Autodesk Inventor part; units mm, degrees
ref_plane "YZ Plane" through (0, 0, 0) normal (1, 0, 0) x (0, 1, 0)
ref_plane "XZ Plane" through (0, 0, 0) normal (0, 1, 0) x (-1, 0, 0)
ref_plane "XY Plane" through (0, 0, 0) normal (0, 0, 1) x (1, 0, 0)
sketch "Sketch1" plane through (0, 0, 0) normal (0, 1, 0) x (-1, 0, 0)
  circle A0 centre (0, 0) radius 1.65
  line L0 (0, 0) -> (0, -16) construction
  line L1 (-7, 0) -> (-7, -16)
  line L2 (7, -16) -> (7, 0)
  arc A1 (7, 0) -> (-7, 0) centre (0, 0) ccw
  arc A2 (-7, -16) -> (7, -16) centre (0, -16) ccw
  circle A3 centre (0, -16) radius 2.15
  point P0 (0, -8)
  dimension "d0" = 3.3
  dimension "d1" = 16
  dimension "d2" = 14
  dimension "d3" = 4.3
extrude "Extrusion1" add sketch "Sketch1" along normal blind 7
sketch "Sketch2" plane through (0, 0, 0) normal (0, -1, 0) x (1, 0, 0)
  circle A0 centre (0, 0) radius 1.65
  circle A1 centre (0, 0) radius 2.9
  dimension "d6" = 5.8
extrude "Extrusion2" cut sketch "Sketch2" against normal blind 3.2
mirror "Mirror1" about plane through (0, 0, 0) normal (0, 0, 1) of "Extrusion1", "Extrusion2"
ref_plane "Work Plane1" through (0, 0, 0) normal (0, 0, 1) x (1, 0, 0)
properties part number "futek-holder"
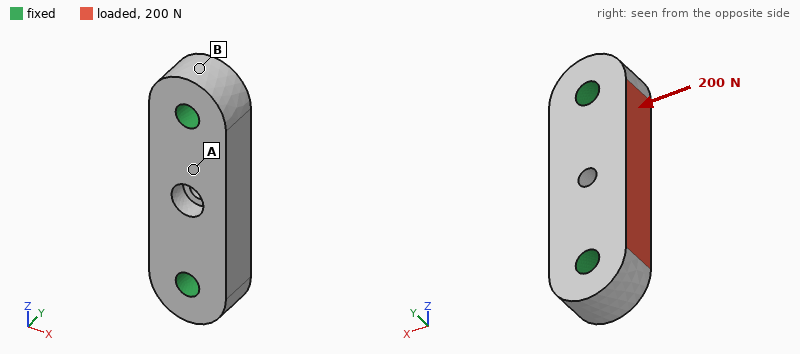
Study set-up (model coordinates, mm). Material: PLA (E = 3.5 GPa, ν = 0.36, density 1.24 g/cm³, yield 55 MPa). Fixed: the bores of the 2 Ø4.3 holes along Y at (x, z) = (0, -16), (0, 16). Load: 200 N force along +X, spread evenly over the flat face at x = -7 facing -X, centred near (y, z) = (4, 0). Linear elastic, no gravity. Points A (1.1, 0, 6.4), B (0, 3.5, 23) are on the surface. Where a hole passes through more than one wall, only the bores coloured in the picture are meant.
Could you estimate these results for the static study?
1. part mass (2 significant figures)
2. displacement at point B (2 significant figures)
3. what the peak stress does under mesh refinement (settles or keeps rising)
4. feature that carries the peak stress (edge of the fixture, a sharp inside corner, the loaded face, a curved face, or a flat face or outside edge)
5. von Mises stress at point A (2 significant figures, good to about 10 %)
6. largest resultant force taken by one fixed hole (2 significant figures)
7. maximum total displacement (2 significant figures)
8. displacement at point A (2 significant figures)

4.8 g
2.3 µm
keeps rising
edge of the fixture
1.1 MPa
100 N
14 µm
9.7 µm
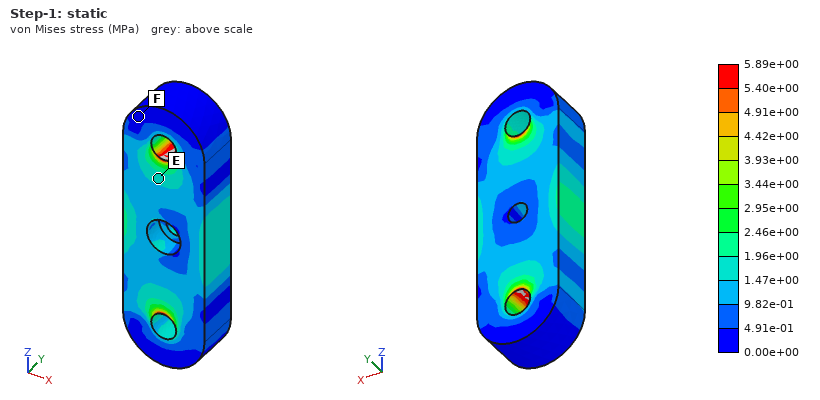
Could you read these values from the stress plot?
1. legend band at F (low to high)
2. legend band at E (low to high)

0.00e+00 to 4.91e-01 MPa
1.47e+00 to 1.96e+00 MPa
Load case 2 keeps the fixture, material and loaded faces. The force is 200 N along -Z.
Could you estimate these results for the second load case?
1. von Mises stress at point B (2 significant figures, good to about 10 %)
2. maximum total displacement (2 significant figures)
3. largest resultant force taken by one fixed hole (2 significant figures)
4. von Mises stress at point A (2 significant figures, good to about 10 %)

0.42 MPa
6.0 µm
110 N
0.58 MPa
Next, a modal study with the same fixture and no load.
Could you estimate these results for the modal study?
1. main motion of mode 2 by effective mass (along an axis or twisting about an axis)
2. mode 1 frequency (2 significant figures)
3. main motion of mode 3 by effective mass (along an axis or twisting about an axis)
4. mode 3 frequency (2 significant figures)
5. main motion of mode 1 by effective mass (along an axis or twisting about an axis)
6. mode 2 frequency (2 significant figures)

along X
9600 Hz
twisting about Z
13 kHz
along Y
12 kHz
